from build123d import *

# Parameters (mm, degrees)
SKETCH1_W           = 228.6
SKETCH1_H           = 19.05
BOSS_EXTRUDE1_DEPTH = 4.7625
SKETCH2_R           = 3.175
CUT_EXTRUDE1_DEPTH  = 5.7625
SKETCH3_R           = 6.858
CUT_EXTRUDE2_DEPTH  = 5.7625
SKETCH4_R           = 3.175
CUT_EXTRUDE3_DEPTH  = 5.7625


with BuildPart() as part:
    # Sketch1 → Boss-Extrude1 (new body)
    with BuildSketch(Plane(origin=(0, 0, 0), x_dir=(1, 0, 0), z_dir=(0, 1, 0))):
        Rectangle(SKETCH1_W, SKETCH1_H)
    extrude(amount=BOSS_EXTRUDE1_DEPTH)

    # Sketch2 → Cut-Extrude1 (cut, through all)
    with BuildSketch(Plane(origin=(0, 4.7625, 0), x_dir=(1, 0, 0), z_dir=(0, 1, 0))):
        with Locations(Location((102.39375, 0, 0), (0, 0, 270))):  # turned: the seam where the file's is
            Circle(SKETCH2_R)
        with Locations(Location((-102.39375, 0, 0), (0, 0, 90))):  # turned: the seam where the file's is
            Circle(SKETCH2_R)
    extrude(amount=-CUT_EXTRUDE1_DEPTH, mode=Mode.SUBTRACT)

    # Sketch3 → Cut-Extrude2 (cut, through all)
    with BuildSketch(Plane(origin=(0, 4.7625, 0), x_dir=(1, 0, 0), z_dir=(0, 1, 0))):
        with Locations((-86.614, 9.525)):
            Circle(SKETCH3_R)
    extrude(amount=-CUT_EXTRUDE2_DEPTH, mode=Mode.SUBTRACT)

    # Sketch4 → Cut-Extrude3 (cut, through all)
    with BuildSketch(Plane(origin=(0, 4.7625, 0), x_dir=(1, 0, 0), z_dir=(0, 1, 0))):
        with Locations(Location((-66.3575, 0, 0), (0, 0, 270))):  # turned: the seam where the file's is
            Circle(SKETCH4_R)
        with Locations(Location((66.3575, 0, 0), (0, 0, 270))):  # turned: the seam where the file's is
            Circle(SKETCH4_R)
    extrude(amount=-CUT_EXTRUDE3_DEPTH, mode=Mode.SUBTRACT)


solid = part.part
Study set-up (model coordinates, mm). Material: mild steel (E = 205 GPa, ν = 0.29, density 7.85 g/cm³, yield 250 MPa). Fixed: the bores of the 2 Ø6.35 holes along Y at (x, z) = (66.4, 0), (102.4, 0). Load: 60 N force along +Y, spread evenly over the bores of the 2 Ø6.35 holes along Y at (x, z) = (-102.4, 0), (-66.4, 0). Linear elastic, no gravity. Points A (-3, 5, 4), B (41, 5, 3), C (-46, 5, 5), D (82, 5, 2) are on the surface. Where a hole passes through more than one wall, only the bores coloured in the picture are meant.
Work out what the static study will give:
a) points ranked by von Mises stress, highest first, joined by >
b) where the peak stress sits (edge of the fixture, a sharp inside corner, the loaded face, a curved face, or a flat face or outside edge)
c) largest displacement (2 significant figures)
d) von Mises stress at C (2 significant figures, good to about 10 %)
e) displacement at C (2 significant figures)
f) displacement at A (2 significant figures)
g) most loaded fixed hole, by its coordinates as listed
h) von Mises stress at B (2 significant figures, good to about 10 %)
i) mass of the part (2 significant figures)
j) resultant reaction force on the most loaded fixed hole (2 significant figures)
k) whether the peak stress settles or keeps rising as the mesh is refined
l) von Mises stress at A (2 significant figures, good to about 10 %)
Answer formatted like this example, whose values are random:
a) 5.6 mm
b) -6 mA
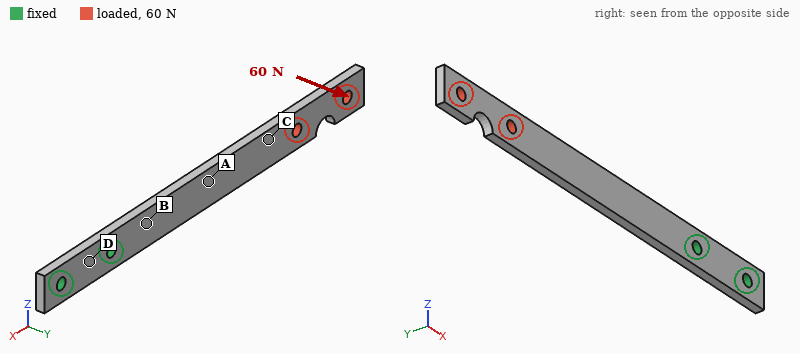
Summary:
a) B > A > C > D
b) edge of the fixture
c) 2.5 mm
d) 32 MPa
e) 1.2 mm
f) 0.49 mm
g) (66.4, 0)
h) 100 MPa
i) 160 g
j) 67 N
k) keeps rising
l) 68 MPa
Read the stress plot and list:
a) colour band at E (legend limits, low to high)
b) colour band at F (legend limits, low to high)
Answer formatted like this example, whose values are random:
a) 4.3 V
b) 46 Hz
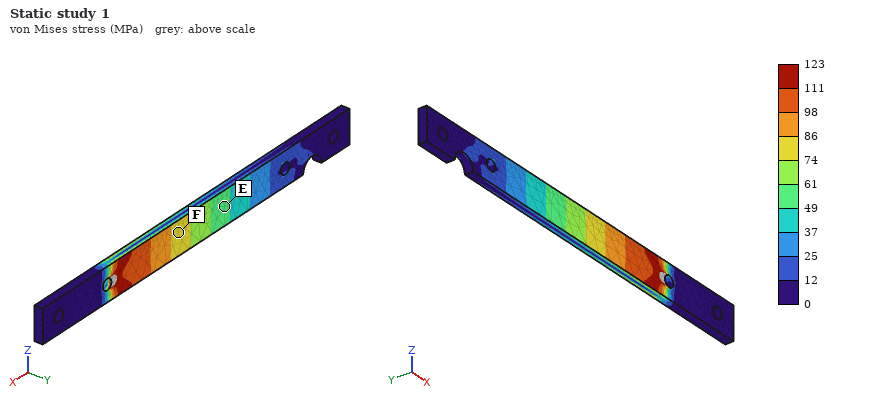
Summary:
a) 49 to 61 MPa
b) 74 to 86 MPa
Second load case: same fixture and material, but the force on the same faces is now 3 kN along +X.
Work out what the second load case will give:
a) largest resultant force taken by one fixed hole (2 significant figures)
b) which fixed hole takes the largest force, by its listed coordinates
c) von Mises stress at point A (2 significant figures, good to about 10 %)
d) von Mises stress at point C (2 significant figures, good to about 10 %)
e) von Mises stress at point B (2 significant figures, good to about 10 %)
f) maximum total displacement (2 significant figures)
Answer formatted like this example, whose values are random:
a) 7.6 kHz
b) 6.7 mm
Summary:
a) 2.8 kN
b) (66.4, 0)
c) 33 MPa
d) 33 MPa
e) 33 MPa
f) 35 µm
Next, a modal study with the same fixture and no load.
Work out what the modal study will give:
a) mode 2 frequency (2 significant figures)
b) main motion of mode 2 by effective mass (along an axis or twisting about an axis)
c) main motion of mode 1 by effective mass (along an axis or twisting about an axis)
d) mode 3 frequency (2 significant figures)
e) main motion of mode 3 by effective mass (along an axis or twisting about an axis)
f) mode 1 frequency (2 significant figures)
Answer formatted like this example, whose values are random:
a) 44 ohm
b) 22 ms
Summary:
a) 480 Hz
b) along Z
c) along Y
d) 770 Hz
e) along Y
f) 130 Hz
